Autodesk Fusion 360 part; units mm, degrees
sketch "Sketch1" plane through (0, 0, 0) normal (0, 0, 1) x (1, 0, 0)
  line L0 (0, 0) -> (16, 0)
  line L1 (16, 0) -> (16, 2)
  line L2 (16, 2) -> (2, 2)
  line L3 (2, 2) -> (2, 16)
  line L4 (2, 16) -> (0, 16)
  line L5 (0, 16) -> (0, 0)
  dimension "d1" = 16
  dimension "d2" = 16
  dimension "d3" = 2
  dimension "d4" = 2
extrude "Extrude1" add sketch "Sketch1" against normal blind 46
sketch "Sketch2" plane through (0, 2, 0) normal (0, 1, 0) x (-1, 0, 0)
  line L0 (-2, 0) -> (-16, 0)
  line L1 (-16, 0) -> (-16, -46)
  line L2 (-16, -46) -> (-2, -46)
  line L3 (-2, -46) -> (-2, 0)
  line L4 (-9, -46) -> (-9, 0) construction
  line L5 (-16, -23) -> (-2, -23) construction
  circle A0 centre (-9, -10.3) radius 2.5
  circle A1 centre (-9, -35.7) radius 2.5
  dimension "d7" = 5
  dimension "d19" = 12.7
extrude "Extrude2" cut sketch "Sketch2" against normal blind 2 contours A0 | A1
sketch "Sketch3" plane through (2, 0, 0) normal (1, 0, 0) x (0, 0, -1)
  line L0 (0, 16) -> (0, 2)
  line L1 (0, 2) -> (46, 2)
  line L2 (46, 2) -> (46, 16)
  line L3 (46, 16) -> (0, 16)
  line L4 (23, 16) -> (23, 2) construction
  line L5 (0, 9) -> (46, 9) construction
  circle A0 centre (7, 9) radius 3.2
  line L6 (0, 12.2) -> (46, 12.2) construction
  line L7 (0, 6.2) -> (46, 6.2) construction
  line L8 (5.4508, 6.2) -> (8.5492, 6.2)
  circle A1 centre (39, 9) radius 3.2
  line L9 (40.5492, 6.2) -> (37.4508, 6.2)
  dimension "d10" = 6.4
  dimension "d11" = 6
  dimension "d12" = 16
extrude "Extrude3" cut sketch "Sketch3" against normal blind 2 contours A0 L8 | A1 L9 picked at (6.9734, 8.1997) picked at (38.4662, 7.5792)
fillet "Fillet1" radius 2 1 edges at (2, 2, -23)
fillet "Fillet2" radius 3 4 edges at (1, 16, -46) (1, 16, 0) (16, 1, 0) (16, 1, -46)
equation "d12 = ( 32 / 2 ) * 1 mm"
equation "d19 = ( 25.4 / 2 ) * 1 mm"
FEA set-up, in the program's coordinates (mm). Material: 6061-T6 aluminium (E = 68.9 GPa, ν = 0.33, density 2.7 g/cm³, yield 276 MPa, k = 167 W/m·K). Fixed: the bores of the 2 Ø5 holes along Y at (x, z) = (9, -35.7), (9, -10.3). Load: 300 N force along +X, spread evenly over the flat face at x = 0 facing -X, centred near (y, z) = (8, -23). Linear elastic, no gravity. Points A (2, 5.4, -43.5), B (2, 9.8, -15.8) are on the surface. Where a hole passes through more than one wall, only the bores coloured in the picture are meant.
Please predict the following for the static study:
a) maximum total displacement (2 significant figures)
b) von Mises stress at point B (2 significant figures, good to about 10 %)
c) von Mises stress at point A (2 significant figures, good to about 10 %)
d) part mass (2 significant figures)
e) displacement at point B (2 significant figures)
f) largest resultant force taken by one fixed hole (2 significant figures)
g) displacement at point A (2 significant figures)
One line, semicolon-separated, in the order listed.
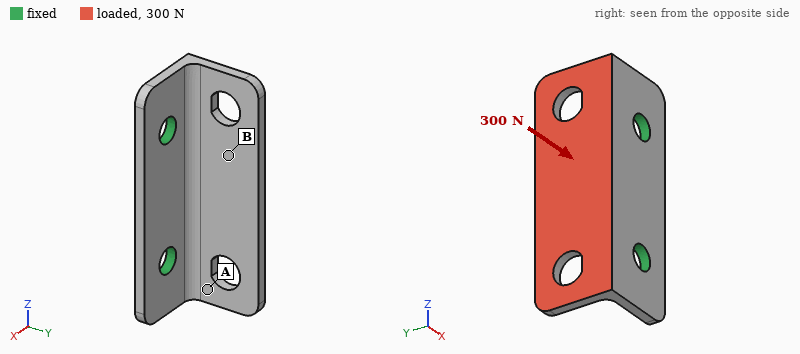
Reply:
0.13 mm; 15 MPa; 38 MPa; 7.0 g; 0.067 mm; 150 N; 0.031 mm
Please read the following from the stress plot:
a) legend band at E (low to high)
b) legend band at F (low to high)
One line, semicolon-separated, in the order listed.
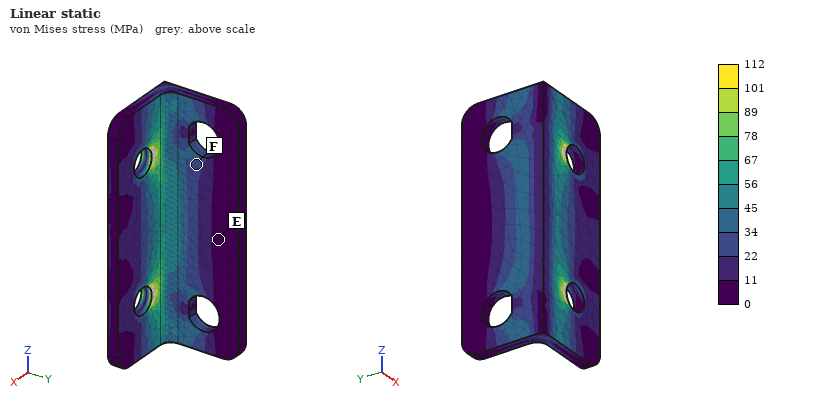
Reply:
0 to 11 MPa; 22 to 34 MPa
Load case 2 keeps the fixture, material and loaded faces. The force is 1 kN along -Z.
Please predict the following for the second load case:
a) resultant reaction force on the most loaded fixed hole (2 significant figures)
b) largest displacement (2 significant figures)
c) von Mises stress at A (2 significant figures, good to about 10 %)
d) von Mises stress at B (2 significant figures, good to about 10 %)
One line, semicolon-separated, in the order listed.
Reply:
620 N; 50 µm; 21 MPa; 21 MPa
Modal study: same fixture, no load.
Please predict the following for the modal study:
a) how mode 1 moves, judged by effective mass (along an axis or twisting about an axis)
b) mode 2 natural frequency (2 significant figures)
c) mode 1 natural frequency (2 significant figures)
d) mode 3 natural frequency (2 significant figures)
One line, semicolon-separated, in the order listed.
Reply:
along X; 6800 Hz; 4700 Hz; 13 kHz
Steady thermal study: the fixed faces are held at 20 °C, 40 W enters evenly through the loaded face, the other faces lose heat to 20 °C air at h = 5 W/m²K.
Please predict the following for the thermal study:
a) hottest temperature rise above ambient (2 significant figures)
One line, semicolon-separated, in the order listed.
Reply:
41 K
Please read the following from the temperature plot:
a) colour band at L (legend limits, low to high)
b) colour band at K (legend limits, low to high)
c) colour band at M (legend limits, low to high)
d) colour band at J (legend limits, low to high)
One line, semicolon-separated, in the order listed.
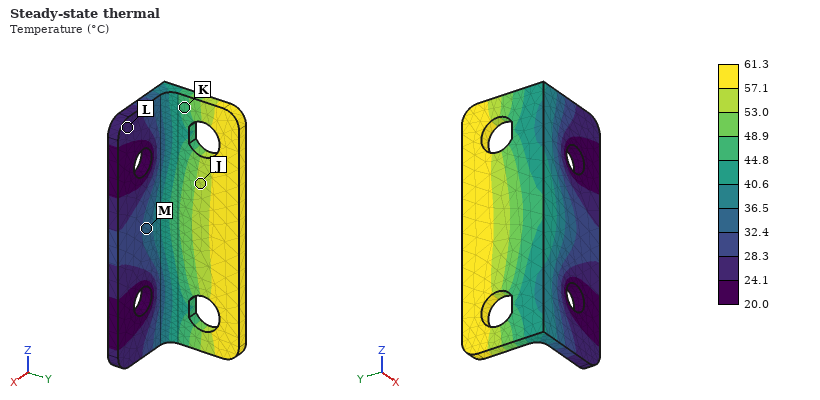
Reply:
24.1 to 28.3 °C; 44.8 to 48.9 °C; 32.4 to 36.5 °C; 53.0 to 57.1 °C
